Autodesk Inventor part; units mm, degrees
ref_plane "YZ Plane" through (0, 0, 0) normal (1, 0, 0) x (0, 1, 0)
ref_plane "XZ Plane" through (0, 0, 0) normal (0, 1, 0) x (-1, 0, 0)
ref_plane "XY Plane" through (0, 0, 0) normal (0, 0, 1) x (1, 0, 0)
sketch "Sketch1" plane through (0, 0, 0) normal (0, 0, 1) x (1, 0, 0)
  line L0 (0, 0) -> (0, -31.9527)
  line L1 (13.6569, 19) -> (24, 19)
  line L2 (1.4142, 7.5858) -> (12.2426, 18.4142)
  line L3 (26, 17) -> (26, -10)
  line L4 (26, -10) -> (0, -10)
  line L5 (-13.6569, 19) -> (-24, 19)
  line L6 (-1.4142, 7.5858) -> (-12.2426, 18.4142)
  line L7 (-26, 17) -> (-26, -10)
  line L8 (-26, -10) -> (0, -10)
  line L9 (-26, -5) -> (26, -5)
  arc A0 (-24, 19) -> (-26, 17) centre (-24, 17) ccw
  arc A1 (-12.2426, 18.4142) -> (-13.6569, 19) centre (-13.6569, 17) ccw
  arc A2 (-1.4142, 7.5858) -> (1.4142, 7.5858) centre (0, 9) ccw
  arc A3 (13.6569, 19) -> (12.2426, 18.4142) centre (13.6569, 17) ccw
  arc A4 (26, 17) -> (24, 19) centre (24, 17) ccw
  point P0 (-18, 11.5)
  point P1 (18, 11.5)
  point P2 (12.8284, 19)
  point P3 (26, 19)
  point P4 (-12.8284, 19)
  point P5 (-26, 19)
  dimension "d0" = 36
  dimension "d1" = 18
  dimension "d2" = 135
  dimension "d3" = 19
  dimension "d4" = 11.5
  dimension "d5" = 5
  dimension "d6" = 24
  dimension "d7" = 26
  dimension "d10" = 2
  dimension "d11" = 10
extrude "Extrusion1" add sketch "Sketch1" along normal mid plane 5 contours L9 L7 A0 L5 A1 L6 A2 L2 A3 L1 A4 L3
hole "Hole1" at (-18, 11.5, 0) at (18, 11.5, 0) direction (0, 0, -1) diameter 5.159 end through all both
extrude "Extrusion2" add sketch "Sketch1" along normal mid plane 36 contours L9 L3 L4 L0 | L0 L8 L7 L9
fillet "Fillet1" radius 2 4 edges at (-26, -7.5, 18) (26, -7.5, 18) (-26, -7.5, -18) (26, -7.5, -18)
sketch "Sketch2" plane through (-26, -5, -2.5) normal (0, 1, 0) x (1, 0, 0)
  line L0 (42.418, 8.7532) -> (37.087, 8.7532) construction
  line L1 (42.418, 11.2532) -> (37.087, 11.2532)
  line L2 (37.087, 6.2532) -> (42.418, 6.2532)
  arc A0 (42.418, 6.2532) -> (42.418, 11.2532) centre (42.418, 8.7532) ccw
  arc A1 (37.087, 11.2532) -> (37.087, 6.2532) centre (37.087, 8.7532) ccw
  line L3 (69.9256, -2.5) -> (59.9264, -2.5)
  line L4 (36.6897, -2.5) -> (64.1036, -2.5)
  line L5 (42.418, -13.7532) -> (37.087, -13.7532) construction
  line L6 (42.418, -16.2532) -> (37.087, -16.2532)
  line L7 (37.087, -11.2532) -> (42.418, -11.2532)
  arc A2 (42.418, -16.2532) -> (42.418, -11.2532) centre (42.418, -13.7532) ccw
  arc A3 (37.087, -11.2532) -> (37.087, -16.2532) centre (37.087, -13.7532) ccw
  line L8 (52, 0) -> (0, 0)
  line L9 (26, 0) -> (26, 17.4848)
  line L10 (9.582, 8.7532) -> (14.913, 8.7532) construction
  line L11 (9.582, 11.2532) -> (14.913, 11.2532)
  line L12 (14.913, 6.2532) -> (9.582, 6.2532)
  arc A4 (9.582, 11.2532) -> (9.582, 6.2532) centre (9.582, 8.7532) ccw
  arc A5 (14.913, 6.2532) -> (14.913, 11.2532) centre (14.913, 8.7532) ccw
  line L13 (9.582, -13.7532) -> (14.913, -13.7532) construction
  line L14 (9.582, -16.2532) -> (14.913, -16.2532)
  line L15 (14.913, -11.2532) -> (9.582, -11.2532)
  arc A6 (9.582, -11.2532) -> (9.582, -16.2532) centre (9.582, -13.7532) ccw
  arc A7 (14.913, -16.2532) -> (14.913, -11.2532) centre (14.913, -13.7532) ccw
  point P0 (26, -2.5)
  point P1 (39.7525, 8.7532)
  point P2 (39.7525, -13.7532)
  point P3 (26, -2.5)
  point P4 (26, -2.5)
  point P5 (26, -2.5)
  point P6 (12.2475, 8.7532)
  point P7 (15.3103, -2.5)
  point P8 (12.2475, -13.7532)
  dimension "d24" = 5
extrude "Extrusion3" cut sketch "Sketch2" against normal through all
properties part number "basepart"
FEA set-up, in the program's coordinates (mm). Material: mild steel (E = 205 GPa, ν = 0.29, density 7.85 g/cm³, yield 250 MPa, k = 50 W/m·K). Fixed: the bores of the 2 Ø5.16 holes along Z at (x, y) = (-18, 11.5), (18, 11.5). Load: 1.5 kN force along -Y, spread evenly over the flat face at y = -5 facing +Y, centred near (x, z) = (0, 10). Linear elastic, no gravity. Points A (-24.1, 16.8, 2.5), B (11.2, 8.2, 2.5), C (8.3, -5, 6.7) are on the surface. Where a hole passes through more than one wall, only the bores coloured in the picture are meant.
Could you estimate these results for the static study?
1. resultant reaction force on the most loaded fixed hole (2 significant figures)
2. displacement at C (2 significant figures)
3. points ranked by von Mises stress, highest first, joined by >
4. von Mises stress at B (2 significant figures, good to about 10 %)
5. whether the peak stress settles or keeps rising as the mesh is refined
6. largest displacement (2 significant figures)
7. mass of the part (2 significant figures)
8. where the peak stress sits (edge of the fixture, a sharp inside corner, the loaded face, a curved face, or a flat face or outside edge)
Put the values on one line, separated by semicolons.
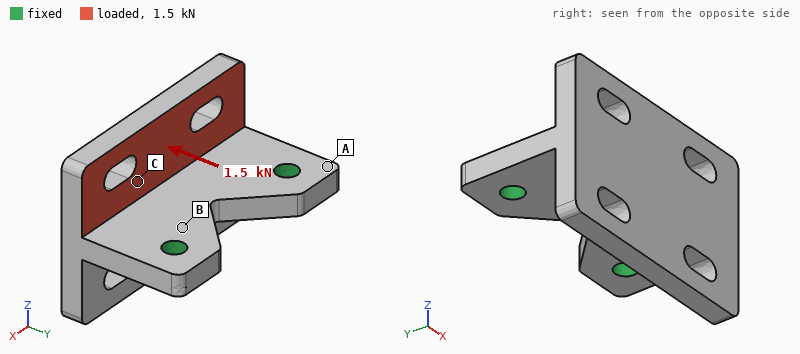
790 N; 28 µm; B > C > A; 67 MPa; keeps rising; 68 µm; 110 g; edge of the fixture
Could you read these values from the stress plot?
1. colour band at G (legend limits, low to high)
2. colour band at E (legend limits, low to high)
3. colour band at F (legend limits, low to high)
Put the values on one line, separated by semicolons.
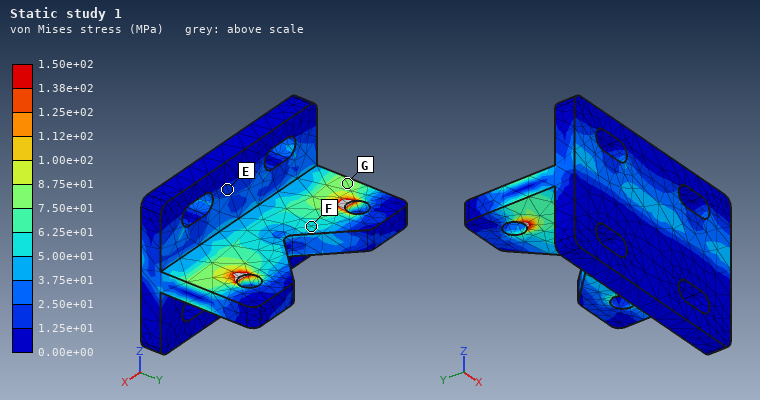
7.50e+01 to 8.75e+01 MPa; 1.25e+01 to 2.50e+01 MPa; 5.00e+01 to 6.25e+01 MPa
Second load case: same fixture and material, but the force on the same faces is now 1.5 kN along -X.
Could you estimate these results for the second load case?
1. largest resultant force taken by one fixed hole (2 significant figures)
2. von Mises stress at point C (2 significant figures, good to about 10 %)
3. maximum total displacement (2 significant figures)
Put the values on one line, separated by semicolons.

1.0 kN; 26 MPa; 20 µm
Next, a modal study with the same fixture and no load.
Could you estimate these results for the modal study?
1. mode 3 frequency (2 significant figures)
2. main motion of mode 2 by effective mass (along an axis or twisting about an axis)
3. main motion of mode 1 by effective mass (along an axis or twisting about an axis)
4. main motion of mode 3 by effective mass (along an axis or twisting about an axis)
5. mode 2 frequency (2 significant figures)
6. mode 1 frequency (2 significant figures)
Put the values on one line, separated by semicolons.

9600 Hz; twisting about Y; along Z; along Z; 5700 Hz; 3000 Hz
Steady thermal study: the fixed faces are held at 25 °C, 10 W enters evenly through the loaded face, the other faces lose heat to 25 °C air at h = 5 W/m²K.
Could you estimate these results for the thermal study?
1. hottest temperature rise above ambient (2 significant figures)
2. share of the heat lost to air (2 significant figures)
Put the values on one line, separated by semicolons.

25 K; 4.2 %
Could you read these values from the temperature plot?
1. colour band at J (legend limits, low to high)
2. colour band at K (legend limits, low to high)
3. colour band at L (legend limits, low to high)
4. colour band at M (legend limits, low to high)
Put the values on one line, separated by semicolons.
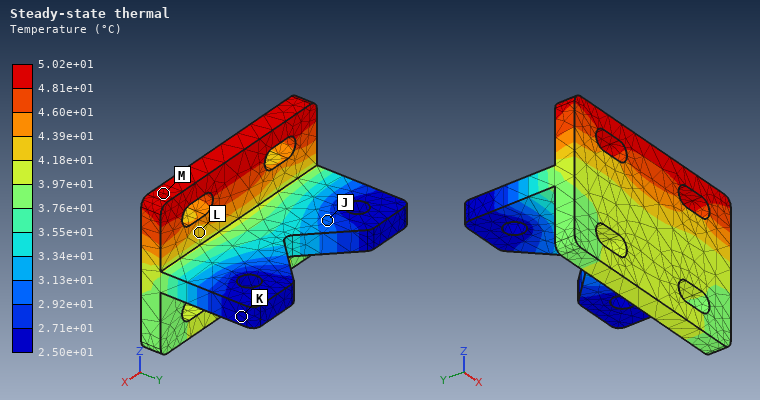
2.92e+01 to 3.13e+01 °C; 2.50e+01 to 2.71e+01 °C; 4.18e+01 to 4.39e+01 °C; 4.81e+01 to 5.02e+01 °C
